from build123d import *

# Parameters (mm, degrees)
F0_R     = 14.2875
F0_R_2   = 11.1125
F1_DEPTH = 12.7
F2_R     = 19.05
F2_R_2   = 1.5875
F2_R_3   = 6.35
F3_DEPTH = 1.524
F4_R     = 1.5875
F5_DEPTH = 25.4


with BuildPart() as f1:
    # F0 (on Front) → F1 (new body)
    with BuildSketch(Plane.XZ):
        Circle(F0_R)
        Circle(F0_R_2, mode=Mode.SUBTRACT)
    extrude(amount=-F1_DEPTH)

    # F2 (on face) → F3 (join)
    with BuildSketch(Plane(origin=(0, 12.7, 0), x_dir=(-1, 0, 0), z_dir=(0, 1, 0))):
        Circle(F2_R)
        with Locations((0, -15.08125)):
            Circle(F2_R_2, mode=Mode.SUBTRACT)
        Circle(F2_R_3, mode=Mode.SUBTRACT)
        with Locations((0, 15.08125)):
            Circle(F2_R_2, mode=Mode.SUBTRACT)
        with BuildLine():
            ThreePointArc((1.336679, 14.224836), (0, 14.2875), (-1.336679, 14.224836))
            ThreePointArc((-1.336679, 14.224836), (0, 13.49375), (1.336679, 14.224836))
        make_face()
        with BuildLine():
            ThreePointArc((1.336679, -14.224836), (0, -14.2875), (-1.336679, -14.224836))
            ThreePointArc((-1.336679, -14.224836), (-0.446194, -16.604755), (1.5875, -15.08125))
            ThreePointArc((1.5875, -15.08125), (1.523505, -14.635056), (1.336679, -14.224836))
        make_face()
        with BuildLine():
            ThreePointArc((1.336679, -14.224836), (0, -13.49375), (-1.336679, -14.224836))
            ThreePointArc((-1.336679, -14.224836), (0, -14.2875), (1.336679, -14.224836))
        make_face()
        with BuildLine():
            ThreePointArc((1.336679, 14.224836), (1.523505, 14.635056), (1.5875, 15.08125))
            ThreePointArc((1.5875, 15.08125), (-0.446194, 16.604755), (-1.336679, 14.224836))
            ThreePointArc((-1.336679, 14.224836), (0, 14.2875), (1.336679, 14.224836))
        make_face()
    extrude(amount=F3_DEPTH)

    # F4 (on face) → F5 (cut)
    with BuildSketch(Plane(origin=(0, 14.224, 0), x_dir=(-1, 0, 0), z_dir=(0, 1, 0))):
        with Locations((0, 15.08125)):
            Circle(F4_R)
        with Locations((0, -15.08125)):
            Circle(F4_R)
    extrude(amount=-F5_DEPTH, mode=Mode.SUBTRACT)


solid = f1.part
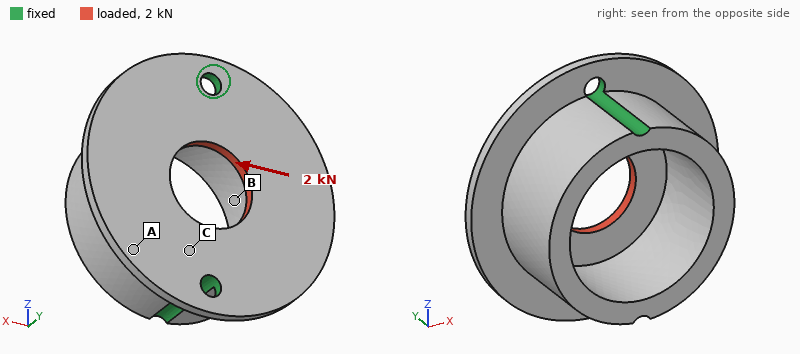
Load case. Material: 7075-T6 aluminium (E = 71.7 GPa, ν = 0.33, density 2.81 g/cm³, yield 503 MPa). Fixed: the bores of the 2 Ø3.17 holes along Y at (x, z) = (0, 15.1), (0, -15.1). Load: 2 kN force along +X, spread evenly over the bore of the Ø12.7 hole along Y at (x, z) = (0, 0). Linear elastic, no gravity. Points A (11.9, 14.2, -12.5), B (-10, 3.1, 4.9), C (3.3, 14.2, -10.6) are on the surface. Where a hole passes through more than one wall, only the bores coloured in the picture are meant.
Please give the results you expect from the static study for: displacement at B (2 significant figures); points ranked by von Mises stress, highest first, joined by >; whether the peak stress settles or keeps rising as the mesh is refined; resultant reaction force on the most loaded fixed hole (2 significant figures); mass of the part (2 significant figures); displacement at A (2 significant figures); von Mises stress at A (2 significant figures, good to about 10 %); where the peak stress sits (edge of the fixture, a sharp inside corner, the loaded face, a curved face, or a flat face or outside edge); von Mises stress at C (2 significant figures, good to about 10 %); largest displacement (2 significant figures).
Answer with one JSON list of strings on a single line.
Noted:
["2.6 µm", "C > A > B", "keeps rising", "1.0 kN", "13 g", "7.0 µm", "17 MPa", "edge of the fixture", "32 MPa", "13 µm"]
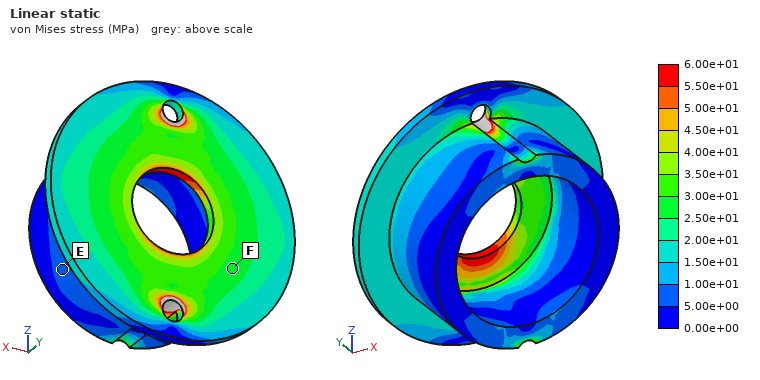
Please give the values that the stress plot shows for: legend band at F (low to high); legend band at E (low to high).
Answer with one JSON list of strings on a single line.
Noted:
["2.50e+01 to 3.00e+01 MPa", "5.00e+00 to 1.00e+01 MPa"]
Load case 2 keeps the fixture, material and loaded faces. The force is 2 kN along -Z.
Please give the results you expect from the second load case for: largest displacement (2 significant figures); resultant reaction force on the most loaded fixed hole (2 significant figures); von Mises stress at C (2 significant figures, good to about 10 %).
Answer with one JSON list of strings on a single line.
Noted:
["8.8 µm", "1.0 kN", "42 MPa"]
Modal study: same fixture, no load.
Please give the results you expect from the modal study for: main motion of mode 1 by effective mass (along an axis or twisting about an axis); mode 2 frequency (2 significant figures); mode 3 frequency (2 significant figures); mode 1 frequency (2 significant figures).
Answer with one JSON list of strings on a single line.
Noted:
["twisting about Z", "22 kHz", "22 kHz", "21 kHz"]
